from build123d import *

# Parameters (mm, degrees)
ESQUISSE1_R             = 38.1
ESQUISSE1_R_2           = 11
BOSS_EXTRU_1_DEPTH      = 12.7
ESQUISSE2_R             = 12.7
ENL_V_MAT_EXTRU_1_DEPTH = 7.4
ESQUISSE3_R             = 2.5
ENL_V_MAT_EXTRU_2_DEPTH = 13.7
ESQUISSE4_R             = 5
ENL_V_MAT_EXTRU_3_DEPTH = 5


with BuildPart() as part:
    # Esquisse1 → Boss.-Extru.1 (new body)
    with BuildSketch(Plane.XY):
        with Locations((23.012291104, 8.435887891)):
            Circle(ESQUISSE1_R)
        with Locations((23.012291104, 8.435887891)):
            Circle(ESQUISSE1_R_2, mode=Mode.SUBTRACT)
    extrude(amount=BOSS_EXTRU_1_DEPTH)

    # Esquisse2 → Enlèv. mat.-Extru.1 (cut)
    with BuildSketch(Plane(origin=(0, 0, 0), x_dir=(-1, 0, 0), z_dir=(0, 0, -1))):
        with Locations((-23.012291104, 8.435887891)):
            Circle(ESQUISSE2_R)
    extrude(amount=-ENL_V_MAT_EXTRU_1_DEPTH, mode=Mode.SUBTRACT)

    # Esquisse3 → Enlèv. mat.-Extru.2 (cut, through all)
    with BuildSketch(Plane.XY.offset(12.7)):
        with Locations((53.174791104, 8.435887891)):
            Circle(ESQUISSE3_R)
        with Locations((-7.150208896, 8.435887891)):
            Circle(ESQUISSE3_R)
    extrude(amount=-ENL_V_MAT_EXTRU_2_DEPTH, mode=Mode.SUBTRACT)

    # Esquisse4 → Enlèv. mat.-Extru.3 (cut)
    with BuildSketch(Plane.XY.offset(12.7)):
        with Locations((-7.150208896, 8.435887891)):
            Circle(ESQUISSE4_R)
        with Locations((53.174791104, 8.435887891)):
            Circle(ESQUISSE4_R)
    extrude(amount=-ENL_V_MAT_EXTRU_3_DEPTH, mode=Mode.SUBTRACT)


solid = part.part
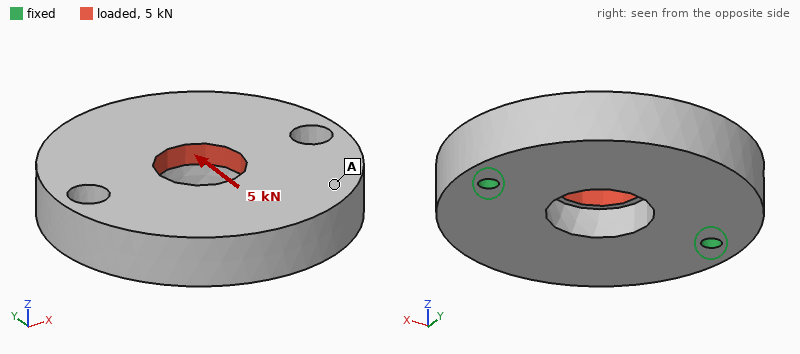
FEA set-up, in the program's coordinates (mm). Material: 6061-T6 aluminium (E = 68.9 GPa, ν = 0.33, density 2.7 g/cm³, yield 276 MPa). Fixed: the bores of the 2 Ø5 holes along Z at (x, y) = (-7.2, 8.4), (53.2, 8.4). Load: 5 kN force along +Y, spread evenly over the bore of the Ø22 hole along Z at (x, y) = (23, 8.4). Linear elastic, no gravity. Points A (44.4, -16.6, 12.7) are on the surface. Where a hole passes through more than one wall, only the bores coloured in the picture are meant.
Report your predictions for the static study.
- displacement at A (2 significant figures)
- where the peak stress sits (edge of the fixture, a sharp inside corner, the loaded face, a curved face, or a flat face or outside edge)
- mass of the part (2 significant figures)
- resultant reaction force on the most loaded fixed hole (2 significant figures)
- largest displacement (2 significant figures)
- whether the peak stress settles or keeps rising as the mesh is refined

29 µm
edge of the fixture
140 g
2.5 kN
45 µm
keeps rising
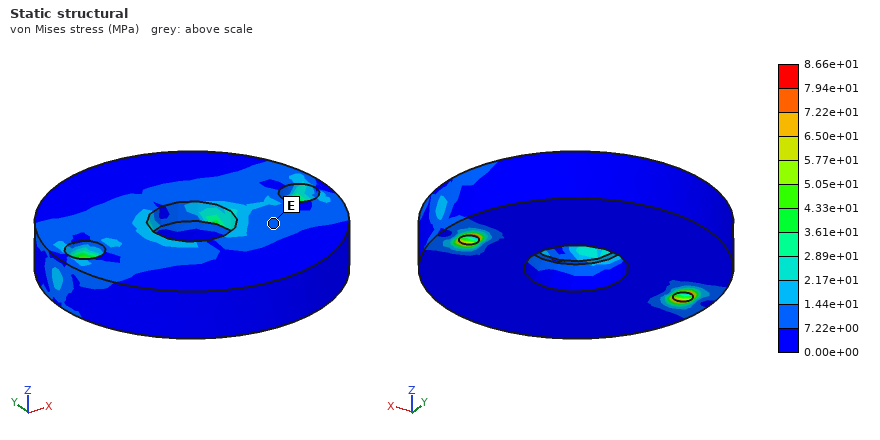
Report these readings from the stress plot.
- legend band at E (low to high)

7.22e+00 to 1.44e+01 MPa
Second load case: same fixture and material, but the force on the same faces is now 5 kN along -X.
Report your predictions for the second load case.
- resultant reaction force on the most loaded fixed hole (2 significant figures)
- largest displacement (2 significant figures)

2.5 kN
6.4 µm
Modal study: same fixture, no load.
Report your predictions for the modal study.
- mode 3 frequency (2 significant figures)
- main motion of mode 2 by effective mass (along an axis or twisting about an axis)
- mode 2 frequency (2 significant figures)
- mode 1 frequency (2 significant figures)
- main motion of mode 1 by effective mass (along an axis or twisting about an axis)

11 kHz
along Z
5800 Hz
3400 Hz
twisting about X
